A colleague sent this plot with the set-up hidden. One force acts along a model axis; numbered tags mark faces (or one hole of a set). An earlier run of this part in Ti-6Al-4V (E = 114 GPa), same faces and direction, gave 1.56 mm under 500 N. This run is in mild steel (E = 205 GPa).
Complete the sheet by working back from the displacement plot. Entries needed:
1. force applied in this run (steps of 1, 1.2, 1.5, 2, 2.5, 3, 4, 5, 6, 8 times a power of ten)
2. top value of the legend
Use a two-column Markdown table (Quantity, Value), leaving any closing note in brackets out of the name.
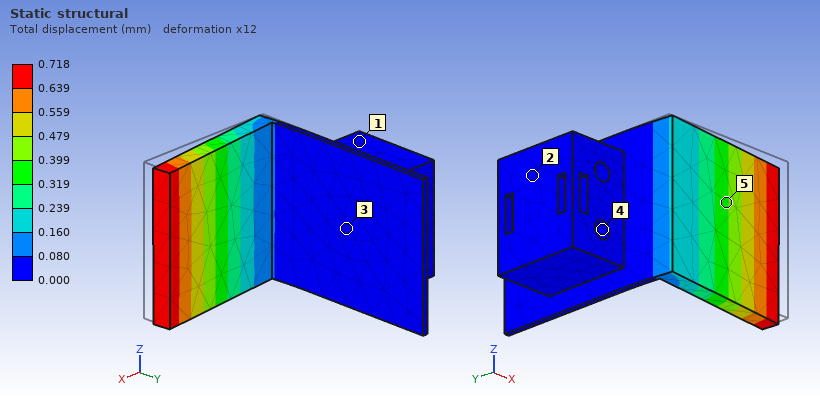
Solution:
| Quantity | Value |
|---|---|
| force applied in this run | 400 N |
| top value of the legend | 0.718 mm |
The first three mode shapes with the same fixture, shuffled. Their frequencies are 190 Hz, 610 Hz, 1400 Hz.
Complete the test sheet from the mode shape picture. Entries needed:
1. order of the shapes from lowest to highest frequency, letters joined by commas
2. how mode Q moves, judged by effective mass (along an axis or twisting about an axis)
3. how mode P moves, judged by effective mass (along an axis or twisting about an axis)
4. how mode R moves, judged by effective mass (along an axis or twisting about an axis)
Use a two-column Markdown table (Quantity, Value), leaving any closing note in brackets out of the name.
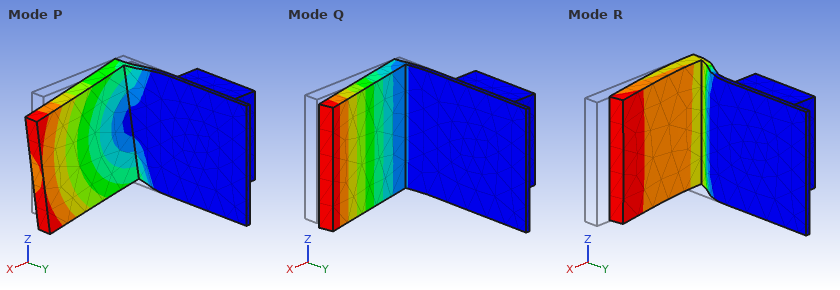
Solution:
| Quantity | Value |
|---|---|
| order of the shapes from lowest to highest frequency, letters joined by commas | Q, P, R |
| how mode Q moves, judged by effective mass | along Y |
| how mode P moves, judged by effective mass | along Z |
| how mode R moves, judged by effective mass | along X |
